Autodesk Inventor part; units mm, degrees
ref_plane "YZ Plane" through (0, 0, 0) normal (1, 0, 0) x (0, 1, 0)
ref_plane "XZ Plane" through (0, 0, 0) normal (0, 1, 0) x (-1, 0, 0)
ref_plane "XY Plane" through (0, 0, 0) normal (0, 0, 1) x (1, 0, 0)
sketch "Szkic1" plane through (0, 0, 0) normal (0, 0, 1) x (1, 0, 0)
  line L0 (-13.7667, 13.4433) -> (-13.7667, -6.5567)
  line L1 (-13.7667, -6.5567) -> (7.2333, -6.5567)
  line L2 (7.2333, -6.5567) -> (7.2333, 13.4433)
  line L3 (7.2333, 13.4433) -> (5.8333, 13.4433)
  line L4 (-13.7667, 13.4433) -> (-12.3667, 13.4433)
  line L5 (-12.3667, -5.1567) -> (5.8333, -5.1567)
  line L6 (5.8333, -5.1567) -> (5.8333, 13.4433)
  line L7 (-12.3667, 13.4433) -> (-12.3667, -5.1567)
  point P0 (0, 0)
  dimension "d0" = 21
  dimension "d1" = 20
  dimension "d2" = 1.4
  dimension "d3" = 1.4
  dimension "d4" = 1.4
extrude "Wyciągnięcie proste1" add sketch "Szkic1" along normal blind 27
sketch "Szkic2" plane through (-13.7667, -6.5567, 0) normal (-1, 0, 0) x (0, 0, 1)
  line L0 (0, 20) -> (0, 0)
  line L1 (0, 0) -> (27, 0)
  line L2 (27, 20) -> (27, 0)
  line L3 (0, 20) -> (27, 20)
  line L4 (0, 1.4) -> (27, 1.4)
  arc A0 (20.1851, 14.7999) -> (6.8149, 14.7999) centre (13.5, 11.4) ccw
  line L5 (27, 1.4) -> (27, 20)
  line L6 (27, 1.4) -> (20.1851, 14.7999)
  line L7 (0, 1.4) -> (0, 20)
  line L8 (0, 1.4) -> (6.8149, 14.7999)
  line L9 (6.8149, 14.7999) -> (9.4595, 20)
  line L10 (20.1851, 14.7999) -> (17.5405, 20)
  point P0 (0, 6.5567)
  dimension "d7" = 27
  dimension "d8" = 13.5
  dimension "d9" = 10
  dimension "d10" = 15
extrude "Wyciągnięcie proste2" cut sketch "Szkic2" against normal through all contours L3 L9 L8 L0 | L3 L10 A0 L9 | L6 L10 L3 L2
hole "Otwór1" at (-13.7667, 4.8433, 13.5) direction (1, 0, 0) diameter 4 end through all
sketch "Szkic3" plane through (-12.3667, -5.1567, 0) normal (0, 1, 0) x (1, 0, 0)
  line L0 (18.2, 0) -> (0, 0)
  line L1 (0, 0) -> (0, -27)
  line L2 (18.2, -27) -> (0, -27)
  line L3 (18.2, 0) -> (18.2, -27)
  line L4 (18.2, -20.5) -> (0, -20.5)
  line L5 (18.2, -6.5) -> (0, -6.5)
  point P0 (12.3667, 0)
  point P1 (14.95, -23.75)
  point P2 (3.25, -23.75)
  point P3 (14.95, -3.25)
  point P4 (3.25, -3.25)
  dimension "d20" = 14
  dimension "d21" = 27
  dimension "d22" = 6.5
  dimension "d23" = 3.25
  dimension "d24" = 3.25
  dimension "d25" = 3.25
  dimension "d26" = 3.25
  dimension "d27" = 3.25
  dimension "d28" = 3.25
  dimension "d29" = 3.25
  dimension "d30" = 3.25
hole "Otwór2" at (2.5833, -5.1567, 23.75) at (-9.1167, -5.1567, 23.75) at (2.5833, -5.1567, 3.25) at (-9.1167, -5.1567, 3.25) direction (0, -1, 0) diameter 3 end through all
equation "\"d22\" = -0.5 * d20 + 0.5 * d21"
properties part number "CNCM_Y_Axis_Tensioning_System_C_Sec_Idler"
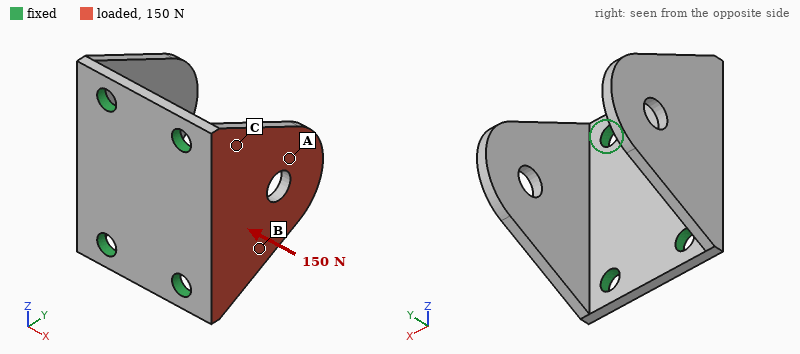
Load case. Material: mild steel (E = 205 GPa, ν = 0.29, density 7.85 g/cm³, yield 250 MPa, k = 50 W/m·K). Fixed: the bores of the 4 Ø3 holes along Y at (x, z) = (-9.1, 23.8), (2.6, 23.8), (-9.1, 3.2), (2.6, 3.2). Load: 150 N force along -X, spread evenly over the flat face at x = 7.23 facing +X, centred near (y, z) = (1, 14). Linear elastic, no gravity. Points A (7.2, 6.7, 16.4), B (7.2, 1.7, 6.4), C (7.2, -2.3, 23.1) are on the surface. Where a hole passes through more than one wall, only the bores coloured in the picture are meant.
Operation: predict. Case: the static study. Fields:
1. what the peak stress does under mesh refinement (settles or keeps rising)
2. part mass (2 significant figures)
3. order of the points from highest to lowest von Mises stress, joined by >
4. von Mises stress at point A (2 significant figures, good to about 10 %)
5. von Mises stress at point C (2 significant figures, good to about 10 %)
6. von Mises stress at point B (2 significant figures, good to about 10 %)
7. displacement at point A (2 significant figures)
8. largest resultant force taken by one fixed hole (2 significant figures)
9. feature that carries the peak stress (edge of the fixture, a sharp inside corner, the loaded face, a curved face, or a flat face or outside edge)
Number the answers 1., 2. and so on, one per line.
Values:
1. keeps rising
2. 12 g
3. C > B > A
4. 18 MPa
5. 82 MPa
6. 51 MPa
7. 0.074 mm
8. 53 N
9. edge of the fixture
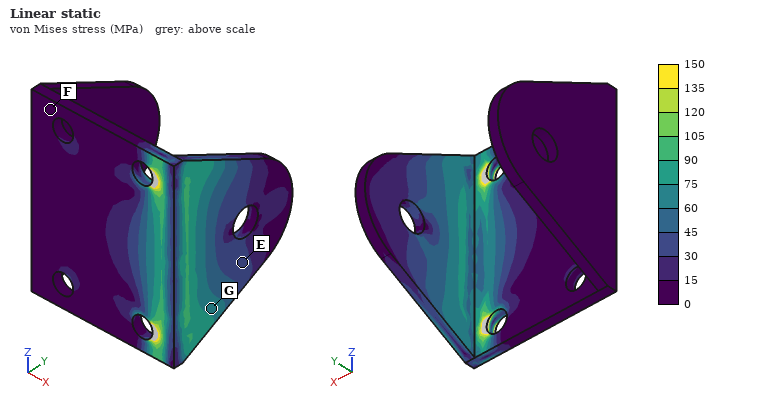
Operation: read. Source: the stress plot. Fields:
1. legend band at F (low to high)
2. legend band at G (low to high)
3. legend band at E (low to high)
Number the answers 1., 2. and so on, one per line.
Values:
1. 0 to 15 MPa
2. 60 to 75 MPa
3. 30 to 45 MPa
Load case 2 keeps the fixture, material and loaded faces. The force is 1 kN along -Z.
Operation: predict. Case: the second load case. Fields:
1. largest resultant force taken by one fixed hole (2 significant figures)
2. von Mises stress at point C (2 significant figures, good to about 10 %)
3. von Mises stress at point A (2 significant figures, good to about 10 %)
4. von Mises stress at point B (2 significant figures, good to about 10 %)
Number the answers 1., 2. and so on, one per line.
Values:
1. 600 N
2. 26 MPa
3. 33 MPa
4. 37 MPa
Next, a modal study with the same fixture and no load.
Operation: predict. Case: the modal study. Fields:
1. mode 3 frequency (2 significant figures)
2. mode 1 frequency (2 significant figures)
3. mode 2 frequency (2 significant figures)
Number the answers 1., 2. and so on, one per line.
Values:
1. 12 kHz
2. 3900 Hz
3. 4000 Hz
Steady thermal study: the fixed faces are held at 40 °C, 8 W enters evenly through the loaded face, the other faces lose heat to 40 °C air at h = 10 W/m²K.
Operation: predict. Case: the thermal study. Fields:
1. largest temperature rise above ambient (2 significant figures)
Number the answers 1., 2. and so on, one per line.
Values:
1. 61 K
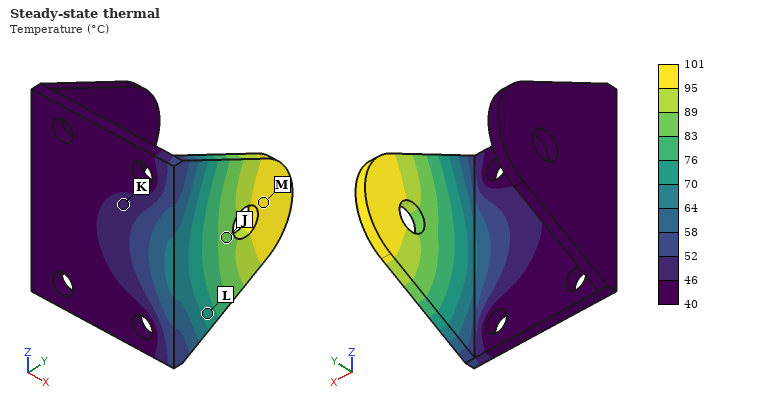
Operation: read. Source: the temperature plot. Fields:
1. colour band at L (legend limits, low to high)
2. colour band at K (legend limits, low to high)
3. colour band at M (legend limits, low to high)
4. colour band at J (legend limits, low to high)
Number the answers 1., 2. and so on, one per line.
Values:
1. 70 to 76 °C
2. 46 to 52 °C
3. 95 to 101 °C
4. 83 to 89 °C
